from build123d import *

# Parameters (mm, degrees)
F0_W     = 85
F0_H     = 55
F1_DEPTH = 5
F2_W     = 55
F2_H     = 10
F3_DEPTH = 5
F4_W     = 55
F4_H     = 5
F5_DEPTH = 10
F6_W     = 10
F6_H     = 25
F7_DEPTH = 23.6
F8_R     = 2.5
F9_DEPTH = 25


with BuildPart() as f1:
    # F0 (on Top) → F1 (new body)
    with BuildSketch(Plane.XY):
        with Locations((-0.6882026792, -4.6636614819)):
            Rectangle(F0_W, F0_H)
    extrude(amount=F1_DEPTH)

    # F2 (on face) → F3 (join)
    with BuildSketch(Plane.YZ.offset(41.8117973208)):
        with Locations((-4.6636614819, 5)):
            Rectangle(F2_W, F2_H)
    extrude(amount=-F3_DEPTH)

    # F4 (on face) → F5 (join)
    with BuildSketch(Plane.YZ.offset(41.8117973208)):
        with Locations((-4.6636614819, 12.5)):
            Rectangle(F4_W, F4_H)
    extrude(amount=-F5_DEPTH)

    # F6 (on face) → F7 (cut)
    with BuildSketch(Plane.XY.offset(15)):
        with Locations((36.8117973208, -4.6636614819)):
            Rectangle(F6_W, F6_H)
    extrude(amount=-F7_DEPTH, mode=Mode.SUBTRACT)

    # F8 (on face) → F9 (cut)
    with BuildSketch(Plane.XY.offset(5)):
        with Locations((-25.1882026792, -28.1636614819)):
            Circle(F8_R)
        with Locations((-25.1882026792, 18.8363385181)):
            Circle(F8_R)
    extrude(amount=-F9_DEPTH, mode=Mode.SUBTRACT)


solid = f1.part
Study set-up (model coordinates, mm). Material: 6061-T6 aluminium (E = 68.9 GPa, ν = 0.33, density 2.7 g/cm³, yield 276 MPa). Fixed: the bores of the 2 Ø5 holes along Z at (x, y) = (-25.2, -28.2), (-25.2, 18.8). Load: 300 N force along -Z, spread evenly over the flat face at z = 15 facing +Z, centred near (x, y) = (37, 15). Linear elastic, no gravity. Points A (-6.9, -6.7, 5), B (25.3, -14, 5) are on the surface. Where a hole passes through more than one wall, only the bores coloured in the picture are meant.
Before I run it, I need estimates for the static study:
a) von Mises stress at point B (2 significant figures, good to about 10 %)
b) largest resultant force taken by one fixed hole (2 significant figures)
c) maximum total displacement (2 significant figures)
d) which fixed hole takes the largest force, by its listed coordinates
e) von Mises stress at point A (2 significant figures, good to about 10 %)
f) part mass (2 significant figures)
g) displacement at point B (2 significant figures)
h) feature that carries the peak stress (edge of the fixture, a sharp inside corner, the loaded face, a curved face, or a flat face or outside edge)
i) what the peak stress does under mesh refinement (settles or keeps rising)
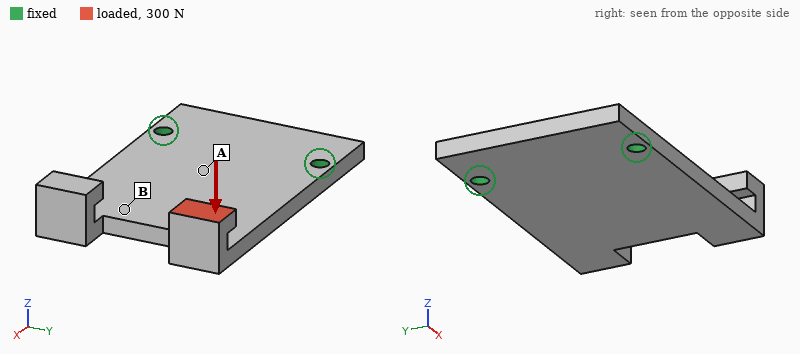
25 MPa
290 N
0.97 mm
(-25.2, 18.8)
53 MPa
65 g
0.46 mm
edge of the fixture
keeps rising
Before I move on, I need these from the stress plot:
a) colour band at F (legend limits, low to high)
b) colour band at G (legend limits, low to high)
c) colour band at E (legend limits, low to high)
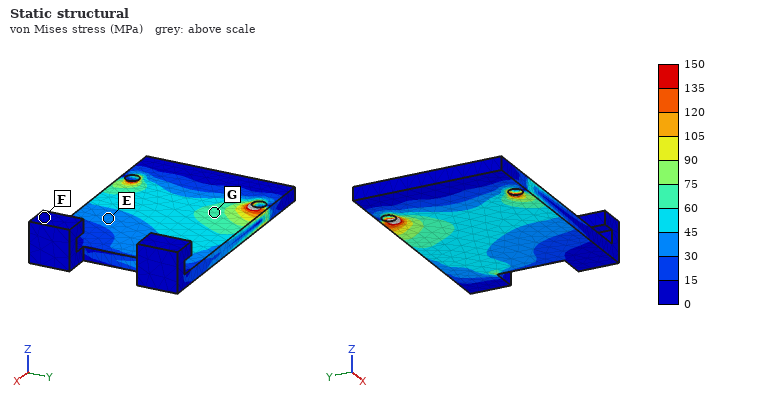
0 to 15 MPa
60 to 75 MPa
30 to 45 MPa
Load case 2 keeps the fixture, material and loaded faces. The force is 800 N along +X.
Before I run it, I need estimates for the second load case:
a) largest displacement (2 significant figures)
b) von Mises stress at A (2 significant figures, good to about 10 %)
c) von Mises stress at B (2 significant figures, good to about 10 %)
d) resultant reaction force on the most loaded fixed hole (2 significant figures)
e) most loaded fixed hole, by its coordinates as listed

0.92 mm
41 MPa
28 MPa
740 N
(-25.2, 18.8)
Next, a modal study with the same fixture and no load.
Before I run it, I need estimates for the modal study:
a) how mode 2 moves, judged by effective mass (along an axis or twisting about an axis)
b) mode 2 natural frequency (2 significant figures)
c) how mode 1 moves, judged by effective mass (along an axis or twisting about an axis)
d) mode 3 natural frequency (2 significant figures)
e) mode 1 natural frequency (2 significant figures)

twisting about X
1900 Hz
along Z
4400 Hz
770 Hz
